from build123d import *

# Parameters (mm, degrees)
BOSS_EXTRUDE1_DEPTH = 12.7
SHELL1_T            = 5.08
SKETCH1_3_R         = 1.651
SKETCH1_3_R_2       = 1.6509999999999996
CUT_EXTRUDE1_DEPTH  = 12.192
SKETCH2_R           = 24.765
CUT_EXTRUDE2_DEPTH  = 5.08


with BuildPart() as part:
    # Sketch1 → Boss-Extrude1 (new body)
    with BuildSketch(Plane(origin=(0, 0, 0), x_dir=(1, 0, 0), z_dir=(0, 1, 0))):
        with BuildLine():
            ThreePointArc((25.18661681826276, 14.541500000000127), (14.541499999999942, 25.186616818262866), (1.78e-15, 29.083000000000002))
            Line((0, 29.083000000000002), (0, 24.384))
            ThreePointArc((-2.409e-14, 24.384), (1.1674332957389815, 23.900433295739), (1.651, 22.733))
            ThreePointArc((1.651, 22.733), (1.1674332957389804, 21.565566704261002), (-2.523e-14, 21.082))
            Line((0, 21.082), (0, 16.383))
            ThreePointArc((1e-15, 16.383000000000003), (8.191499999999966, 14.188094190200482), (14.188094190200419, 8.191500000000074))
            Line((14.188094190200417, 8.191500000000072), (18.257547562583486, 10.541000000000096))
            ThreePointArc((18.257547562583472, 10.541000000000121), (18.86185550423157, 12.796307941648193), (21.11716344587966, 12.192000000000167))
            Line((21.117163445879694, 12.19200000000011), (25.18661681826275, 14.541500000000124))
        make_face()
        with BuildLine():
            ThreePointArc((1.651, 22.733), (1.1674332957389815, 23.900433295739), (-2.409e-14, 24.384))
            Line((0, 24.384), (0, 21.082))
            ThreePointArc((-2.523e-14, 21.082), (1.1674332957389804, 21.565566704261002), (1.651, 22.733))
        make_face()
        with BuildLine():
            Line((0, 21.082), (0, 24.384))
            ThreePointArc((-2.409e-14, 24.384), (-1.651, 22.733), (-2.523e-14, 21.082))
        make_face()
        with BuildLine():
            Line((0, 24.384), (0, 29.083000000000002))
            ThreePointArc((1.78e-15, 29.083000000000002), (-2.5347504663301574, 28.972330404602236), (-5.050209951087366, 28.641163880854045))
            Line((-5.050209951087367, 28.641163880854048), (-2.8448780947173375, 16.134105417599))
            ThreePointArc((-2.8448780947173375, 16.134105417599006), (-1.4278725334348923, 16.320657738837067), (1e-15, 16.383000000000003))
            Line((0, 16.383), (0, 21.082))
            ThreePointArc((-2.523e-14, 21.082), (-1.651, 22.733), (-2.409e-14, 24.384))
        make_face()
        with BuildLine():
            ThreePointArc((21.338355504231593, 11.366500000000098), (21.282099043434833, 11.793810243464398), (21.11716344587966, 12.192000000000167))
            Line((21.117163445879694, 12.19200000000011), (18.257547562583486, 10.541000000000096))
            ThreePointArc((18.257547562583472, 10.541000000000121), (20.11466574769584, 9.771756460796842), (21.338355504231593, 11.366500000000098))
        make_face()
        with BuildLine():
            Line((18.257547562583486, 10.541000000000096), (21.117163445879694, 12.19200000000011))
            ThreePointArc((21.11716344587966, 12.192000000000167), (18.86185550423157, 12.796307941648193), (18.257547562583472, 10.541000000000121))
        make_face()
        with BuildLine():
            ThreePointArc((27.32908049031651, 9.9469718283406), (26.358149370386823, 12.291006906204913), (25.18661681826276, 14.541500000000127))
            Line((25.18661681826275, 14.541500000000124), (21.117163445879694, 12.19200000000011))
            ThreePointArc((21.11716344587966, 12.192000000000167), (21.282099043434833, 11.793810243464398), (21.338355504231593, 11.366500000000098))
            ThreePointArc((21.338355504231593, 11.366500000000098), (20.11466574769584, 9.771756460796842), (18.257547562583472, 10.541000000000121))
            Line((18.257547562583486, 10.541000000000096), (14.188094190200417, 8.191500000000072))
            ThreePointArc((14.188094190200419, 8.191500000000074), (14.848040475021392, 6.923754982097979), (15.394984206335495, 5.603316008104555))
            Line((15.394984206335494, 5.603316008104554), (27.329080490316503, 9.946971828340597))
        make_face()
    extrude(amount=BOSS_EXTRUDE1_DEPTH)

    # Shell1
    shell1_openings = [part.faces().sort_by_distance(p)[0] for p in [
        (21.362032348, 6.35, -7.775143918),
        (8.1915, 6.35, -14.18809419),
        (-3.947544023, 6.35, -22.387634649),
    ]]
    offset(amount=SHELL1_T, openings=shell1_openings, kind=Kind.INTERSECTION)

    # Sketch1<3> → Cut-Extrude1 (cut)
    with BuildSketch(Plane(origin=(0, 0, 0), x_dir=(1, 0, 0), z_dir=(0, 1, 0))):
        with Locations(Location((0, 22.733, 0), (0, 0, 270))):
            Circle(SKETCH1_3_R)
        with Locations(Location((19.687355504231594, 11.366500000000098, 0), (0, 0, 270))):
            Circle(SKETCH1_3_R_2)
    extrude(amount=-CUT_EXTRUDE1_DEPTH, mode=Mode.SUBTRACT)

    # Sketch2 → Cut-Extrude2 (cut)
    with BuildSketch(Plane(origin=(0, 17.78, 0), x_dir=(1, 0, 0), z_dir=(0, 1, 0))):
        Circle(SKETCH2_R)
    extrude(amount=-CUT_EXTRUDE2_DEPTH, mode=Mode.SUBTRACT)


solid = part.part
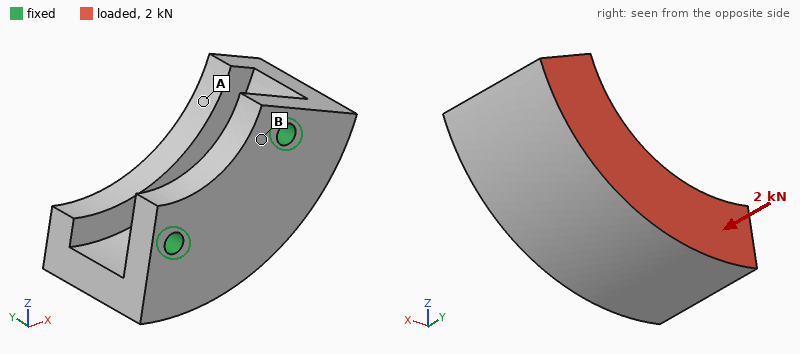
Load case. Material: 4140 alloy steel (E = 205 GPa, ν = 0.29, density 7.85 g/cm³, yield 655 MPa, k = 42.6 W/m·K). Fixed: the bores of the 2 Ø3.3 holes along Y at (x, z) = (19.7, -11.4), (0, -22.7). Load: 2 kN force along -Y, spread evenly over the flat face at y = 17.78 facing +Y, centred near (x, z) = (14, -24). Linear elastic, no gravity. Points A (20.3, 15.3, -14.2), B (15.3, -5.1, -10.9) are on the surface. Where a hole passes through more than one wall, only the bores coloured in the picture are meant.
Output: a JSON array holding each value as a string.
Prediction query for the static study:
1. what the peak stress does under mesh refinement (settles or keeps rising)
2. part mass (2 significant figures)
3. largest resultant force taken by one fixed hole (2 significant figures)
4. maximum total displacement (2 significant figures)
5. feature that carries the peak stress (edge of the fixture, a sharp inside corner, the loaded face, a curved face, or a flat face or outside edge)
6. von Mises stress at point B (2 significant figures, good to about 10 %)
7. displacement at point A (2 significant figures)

["keeps rising", "62 g", "1.0 kN", "20 µm", "edge of the fixture", "35 MPa", "15 µm"]
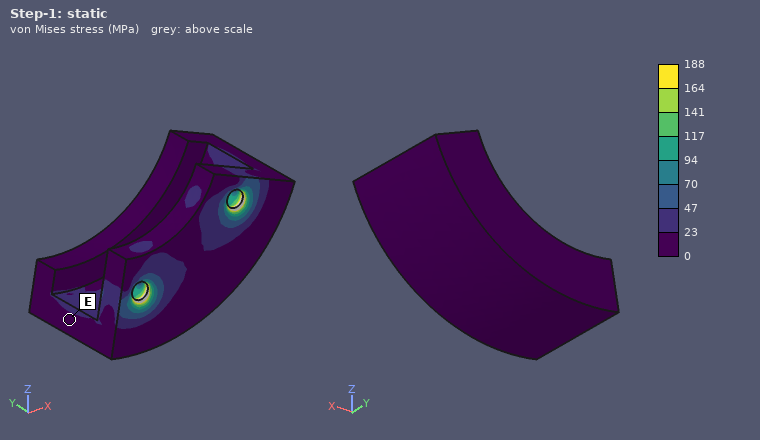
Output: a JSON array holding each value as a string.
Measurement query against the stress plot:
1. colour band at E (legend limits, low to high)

["0 to 23 MPa"]
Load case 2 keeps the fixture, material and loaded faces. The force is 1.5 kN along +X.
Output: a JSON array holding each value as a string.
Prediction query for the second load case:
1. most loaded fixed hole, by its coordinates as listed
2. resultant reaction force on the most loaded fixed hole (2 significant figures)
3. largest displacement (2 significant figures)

["(0, -22.7)", "1.4 kN", "68 µm"]
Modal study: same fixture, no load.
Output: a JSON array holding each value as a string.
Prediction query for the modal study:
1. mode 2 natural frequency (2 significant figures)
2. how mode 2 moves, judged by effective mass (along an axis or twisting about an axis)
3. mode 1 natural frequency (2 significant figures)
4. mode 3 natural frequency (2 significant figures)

["8100 Hz", "along X", "4500 Hz", "14 kHz"]
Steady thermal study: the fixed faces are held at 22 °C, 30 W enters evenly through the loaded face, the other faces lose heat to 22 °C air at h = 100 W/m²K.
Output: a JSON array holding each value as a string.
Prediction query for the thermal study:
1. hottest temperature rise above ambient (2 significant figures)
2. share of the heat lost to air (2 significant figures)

["70 K", "38 %"]
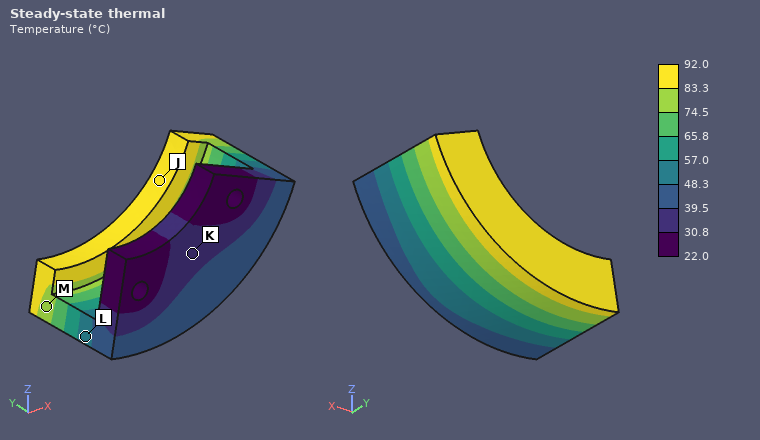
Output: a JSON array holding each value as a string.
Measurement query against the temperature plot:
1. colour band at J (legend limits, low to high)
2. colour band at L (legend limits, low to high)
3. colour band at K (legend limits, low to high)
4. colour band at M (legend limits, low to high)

["83.3 to 92.0 °C", "48.3 to 57.0 °C", "30.8 to 39.5 °C", "74.5 to 83.3 °C"]
